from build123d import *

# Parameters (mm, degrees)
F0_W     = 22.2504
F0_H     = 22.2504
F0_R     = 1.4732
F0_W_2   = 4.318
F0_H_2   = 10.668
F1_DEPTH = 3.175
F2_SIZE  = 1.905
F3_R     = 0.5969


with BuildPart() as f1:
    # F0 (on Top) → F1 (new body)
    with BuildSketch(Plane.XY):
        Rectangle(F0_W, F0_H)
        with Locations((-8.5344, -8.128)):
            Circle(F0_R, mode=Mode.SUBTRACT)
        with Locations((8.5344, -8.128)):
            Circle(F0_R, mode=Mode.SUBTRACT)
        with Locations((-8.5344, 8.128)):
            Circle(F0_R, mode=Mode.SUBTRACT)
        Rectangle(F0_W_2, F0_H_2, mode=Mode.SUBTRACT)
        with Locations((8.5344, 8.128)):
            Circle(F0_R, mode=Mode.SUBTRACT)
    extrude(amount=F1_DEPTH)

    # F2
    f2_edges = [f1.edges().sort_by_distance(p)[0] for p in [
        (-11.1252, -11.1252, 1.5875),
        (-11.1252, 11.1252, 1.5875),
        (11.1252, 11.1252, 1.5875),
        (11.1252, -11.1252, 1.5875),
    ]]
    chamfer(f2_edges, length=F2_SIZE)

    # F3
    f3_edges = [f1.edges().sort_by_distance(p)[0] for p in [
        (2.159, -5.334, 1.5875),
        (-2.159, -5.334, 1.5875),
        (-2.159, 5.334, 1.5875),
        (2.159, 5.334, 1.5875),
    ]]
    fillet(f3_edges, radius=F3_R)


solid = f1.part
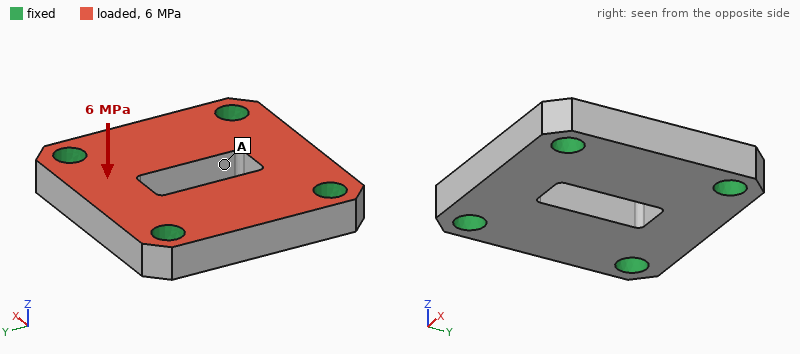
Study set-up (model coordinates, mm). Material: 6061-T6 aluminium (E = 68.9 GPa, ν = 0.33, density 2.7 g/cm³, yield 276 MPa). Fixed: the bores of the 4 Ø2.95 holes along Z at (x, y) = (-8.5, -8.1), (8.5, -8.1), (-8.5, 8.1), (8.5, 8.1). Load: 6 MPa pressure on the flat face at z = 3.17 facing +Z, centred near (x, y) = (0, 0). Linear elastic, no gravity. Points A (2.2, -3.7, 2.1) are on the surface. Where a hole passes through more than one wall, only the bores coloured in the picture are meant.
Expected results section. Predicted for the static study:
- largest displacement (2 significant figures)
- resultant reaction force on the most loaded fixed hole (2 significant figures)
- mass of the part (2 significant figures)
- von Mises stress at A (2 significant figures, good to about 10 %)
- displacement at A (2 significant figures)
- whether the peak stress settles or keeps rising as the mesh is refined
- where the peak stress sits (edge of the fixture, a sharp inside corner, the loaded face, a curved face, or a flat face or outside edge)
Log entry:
16 µm
620 N
3.6 g
20 MPa
13 µm
keeps rising
edge of the fixture
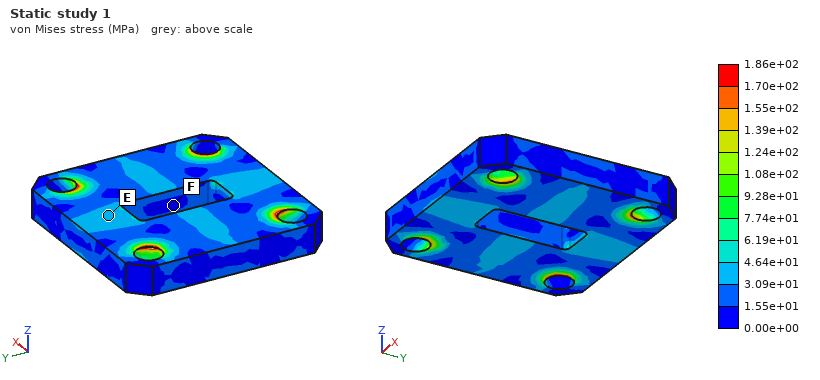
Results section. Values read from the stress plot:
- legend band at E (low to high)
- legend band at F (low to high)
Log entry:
3.09e+01 to 4.64e+01 MPa
0.00e+00 to 1.55e+01 MPa
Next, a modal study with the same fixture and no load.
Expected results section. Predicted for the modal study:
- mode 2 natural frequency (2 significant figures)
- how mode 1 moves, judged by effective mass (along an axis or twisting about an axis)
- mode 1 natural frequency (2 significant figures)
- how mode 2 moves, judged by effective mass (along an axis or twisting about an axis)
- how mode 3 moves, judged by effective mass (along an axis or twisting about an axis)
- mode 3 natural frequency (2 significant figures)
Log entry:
56 kHz
along Z
44 kHz
twisting about Y
twisting about X
60 kHz
